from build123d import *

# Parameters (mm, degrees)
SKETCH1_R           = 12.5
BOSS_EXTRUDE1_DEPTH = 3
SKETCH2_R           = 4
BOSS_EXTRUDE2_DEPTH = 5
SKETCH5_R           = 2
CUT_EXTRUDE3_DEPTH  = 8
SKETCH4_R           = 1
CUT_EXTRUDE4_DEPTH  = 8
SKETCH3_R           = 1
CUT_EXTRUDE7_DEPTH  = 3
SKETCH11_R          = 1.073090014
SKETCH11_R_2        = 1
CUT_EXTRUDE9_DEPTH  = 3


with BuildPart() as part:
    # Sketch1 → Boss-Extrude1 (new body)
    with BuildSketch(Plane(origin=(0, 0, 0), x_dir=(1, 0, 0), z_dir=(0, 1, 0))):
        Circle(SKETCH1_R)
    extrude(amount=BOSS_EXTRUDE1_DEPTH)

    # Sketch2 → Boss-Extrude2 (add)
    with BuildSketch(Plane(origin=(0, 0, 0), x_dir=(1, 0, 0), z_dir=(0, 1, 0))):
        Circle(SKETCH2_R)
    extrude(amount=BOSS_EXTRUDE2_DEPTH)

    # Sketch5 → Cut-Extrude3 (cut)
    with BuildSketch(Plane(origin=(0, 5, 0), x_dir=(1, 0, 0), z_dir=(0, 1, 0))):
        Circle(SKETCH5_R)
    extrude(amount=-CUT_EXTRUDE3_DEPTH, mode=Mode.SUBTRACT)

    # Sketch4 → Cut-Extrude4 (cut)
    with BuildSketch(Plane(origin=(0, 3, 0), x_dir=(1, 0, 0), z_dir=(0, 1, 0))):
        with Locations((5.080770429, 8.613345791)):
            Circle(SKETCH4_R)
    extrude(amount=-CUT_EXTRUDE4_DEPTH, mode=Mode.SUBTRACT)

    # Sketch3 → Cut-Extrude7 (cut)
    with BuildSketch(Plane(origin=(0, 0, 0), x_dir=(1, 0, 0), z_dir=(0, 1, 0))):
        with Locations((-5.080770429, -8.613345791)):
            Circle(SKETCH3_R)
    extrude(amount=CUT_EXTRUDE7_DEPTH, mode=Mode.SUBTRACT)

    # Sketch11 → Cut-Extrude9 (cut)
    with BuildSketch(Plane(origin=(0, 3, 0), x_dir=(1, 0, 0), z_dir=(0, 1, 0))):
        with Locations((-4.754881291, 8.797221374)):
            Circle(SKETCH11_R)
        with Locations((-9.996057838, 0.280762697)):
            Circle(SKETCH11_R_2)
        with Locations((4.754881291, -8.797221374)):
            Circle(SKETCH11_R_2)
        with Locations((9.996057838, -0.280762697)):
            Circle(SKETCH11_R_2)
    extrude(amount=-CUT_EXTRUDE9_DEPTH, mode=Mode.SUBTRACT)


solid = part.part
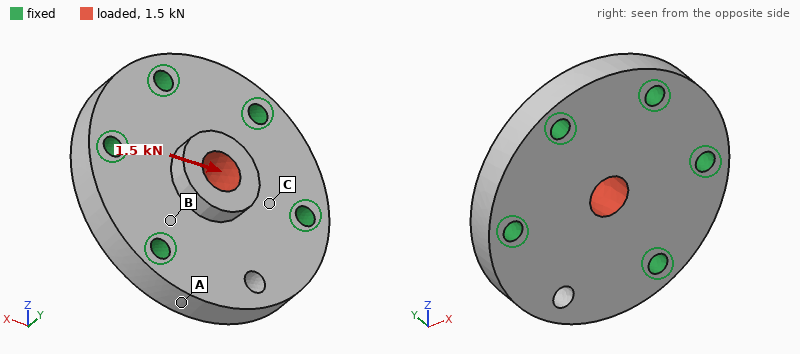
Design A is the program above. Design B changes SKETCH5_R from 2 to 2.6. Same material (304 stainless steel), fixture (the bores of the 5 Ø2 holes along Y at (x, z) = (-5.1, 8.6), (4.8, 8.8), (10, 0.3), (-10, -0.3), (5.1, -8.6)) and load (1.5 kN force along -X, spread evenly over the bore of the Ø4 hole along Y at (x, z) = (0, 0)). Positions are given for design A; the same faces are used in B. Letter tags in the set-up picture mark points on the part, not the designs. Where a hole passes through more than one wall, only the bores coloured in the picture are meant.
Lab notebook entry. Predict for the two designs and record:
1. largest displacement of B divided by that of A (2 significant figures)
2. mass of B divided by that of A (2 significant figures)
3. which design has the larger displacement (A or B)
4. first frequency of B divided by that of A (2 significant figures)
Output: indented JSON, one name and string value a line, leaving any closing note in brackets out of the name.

{
  "largest displacement of B divided by that of A": "1.1",
  "mass of B divided by that of A": "0.97",
  "which design has the larger displacement": "B",
  "first frequency of B divided by that of A": "0.99"
}
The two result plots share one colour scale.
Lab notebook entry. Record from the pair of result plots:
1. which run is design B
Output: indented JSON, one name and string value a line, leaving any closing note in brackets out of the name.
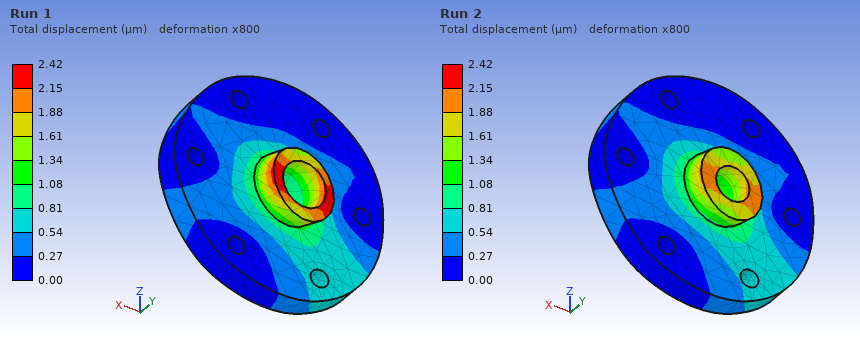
{
  "which run is design B": "Run 1"
}
